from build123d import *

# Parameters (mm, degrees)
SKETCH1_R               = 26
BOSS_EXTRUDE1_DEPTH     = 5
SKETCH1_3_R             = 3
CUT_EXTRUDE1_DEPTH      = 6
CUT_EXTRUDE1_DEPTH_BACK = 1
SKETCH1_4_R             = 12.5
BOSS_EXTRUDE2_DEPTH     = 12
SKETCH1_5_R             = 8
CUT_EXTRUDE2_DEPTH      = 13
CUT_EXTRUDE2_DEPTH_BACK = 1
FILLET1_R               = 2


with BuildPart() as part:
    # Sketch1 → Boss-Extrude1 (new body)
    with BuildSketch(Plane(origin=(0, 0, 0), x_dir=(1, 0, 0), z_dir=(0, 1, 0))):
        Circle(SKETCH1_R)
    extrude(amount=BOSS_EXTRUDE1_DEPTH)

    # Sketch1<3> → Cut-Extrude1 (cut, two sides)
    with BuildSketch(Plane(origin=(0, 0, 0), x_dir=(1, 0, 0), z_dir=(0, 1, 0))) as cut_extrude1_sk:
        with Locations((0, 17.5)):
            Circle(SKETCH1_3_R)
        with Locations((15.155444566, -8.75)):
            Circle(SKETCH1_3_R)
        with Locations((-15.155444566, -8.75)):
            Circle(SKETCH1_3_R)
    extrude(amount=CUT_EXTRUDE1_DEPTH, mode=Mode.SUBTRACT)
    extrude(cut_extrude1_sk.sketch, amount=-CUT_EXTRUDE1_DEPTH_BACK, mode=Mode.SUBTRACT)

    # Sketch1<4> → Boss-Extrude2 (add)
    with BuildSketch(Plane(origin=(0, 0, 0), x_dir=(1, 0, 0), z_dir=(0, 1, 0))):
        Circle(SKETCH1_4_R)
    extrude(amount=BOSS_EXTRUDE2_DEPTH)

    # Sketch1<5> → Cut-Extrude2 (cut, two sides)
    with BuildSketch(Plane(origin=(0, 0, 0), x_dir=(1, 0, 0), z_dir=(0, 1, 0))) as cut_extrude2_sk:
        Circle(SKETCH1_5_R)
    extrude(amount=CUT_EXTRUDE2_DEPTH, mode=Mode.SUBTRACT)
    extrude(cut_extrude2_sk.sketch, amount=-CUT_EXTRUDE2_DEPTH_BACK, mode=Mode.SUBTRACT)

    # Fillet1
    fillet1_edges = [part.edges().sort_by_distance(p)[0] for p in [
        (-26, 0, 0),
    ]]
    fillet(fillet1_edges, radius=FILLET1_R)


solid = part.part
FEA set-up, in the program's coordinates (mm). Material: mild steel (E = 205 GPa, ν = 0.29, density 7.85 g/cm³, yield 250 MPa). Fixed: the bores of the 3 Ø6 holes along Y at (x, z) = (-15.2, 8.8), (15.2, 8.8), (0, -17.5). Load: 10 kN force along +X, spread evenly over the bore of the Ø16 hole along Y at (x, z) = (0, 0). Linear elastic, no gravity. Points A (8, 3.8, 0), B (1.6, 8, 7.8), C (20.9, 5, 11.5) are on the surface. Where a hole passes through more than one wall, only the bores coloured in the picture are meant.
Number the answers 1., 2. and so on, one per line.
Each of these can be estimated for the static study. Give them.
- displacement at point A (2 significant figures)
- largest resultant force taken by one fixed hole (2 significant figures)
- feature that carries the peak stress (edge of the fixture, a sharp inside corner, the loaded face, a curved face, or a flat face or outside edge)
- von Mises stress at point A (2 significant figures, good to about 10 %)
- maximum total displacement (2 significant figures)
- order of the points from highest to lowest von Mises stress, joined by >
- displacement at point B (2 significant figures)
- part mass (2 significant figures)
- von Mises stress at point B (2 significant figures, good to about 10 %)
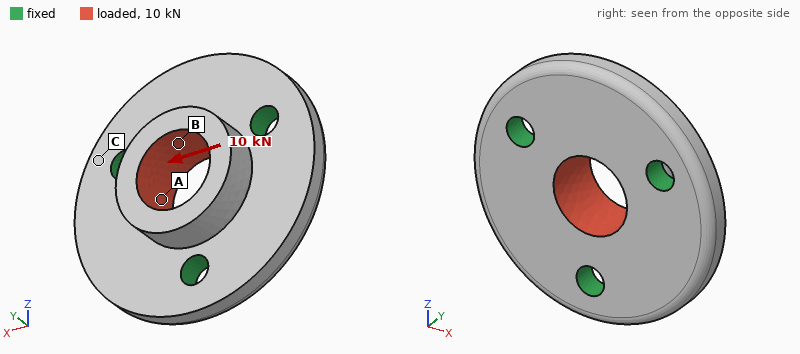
1. 3.0 µm
2. 3.5 kN
3. edge of the fixture
4. 33 MPa
5. 7.9 µm
6. B > A > C
7. 3.2 µm
8. 87 g
9. 52 MPa
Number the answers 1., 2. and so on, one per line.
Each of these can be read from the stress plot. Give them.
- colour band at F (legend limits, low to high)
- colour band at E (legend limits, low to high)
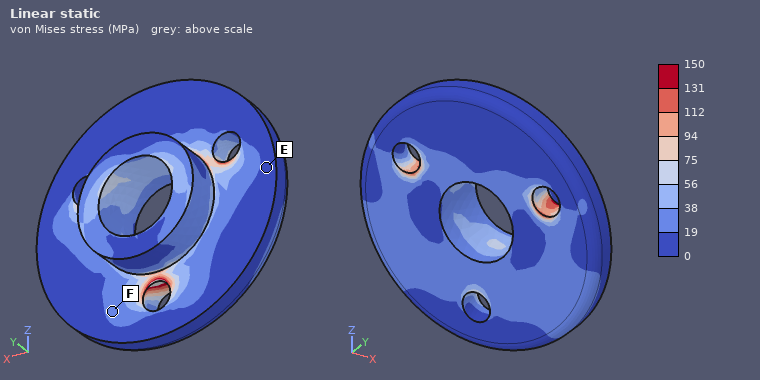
1. 19 to 38 MPa
2. 0 to 19 MPa
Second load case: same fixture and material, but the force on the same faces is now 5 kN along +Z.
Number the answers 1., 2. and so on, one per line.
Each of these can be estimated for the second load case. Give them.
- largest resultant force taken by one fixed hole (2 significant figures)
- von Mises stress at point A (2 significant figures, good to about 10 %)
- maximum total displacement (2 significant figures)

1. 1.7 kN
2. 22 MPa
3. 4.4 µm
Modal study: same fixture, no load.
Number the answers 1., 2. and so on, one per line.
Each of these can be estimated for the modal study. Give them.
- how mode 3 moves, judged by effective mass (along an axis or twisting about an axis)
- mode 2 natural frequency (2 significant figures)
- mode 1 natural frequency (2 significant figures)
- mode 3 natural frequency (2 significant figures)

1. along Y
2. 16 kHz
3. 16 kHz
4. 18 kHz
